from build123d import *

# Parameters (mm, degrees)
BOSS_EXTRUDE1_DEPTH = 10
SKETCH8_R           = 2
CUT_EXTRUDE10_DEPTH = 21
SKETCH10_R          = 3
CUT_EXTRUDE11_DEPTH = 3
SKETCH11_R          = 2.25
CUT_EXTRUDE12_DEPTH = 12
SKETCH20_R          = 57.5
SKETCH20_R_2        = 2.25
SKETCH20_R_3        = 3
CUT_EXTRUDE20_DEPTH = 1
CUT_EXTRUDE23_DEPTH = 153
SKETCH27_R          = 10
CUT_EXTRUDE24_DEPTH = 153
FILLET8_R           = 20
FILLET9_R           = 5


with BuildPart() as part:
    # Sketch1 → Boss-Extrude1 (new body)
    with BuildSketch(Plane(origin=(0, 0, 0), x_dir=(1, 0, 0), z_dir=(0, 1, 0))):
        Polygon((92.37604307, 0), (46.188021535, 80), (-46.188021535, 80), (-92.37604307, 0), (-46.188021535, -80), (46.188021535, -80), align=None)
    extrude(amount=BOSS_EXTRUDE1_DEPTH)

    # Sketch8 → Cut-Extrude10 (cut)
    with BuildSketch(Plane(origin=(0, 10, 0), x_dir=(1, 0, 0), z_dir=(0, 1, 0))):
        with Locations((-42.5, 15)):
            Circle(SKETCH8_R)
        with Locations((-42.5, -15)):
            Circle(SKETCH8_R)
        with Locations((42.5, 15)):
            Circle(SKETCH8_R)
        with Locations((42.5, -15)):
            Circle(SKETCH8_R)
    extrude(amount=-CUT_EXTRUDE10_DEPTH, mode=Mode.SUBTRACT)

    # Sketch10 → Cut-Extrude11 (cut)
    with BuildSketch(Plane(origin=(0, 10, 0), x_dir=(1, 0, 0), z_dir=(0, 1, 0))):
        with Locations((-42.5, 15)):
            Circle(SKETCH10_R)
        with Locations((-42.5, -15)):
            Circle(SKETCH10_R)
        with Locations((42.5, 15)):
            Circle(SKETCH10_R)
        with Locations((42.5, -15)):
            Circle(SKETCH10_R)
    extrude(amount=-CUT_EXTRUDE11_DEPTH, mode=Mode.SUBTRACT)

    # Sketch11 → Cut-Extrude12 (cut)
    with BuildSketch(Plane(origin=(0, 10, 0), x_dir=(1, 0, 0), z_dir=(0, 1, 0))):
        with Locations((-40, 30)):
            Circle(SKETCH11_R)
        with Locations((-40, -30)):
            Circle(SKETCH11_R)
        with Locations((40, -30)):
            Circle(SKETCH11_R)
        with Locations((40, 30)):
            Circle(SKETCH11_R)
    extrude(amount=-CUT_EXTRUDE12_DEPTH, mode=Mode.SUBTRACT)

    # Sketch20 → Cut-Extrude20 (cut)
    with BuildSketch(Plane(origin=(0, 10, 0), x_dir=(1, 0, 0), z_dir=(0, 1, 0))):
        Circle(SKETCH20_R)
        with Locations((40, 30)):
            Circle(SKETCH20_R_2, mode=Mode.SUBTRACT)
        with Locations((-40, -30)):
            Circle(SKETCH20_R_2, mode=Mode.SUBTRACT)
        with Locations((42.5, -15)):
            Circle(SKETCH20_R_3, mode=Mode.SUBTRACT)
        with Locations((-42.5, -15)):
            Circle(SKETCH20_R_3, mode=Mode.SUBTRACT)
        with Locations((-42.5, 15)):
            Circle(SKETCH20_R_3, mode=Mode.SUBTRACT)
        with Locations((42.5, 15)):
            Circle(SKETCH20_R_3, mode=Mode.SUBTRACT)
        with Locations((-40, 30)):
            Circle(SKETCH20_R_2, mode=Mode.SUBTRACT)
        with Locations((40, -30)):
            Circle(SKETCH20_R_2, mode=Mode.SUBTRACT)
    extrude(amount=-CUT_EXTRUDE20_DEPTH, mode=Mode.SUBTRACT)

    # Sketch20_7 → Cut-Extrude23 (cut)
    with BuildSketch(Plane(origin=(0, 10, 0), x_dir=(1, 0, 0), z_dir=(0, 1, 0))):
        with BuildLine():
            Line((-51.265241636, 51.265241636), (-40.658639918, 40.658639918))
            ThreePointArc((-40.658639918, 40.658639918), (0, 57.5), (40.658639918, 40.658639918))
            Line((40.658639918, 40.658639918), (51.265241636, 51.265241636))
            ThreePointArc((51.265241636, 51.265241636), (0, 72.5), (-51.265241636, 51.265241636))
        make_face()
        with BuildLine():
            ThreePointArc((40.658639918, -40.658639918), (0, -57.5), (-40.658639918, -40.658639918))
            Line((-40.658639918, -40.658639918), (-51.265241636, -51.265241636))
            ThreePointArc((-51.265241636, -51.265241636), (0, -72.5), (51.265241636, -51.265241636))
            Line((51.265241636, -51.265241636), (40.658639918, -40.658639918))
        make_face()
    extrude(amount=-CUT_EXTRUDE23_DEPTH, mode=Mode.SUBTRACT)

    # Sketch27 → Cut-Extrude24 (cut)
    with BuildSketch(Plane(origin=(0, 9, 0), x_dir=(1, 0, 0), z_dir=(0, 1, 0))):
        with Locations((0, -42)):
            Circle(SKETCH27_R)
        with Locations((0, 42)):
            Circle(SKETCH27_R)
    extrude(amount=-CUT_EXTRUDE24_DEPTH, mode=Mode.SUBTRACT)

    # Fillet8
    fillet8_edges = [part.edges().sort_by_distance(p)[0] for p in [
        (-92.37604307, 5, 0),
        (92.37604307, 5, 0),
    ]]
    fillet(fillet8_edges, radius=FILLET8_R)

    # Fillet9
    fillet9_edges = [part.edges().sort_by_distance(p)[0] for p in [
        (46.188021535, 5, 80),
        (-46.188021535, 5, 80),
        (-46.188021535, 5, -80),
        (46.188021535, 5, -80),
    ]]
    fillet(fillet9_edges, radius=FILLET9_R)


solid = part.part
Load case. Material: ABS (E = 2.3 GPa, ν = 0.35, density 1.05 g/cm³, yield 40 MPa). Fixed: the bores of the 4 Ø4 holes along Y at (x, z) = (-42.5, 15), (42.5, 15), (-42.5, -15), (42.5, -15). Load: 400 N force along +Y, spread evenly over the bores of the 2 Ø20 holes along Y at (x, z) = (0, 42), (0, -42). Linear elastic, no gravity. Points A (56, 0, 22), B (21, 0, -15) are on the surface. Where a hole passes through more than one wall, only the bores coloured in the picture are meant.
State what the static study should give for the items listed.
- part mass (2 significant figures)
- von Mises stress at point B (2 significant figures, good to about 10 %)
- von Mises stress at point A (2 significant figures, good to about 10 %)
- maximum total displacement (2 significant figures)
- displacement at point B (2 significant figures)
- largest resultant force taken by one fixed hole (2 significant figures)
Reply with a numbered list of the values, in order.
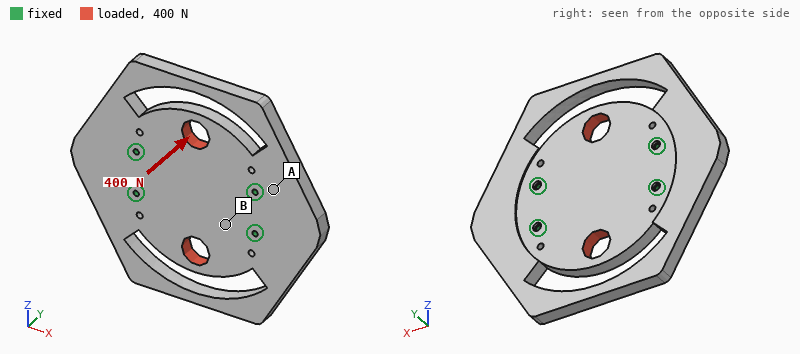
1. 180 g
2. 2.8 MPa
3. 1.3 MPa
4. 0.57 mm
5. 0.11 mm
6. 120 N
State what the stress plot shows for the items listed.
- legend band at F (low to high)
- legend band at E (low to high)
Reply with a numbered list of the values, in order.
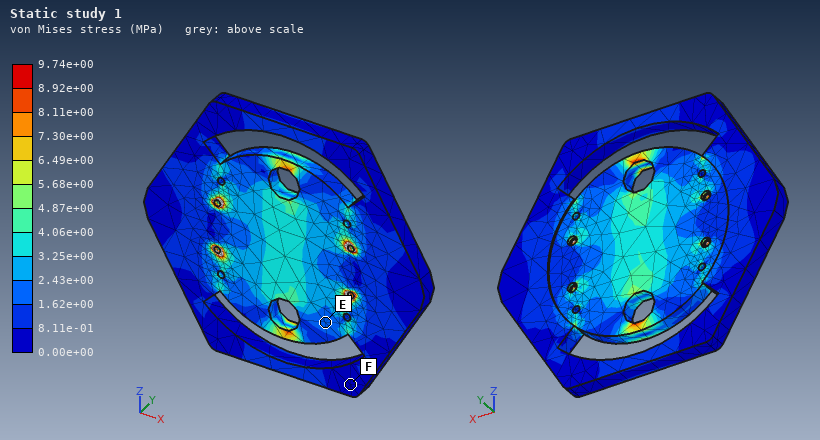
1. 0.00e+00 to 8.11e-01 MPa
2. 1.62e+00 to 2.43e+00 MPa
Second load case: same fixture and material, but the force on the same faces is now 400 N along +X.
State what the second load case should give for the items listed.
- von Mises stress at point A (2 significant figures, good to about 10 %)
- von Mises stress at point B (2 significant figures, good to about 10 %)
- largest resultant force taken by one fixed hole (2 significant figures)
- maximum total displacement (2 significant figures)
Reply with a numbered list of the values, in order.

1. 0.24 MPa
2. 0.24 MPa
3. 100 N
4. 17 µm
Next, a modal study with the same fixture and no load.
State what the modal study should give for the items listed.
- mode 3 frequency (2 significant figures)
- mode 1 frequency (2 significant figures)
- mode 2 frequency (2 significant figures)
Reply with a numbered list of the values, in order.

1. 750 Hz
2. 430 Hz
3. 430 Hz
